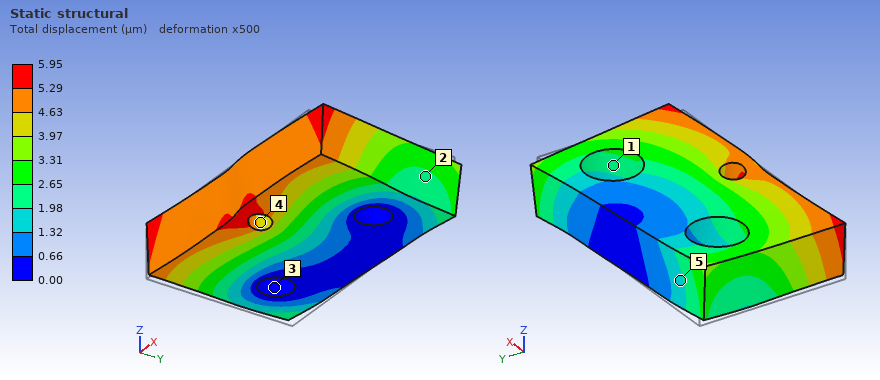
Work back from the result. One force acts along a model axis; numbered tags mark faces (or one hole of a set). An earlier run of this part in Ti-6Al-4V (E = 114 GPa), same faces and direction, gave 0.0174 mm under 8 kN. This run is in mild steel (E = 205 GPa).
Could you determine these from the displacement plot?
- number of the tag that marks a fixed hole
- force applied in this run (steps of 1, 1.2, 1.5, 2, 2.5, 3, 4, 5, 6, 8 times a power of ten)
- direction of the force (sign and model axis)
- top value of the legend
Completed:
3
5 kN
+X
5.95 µm
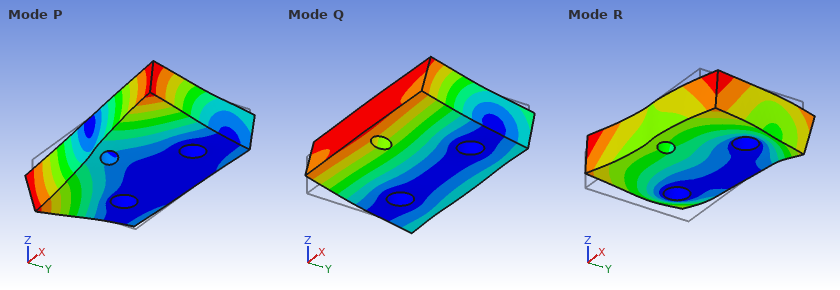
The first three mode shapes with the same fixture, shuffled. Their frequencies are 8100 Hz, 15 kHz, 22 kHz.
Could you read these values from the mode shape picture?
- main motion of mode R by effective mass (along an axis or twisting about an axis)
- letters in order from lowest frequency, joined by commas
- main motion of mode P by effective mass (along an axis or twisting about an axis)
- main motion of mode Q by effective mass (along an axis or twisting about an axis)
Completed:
along X
Q, P, R
twisting about Y
along Z
